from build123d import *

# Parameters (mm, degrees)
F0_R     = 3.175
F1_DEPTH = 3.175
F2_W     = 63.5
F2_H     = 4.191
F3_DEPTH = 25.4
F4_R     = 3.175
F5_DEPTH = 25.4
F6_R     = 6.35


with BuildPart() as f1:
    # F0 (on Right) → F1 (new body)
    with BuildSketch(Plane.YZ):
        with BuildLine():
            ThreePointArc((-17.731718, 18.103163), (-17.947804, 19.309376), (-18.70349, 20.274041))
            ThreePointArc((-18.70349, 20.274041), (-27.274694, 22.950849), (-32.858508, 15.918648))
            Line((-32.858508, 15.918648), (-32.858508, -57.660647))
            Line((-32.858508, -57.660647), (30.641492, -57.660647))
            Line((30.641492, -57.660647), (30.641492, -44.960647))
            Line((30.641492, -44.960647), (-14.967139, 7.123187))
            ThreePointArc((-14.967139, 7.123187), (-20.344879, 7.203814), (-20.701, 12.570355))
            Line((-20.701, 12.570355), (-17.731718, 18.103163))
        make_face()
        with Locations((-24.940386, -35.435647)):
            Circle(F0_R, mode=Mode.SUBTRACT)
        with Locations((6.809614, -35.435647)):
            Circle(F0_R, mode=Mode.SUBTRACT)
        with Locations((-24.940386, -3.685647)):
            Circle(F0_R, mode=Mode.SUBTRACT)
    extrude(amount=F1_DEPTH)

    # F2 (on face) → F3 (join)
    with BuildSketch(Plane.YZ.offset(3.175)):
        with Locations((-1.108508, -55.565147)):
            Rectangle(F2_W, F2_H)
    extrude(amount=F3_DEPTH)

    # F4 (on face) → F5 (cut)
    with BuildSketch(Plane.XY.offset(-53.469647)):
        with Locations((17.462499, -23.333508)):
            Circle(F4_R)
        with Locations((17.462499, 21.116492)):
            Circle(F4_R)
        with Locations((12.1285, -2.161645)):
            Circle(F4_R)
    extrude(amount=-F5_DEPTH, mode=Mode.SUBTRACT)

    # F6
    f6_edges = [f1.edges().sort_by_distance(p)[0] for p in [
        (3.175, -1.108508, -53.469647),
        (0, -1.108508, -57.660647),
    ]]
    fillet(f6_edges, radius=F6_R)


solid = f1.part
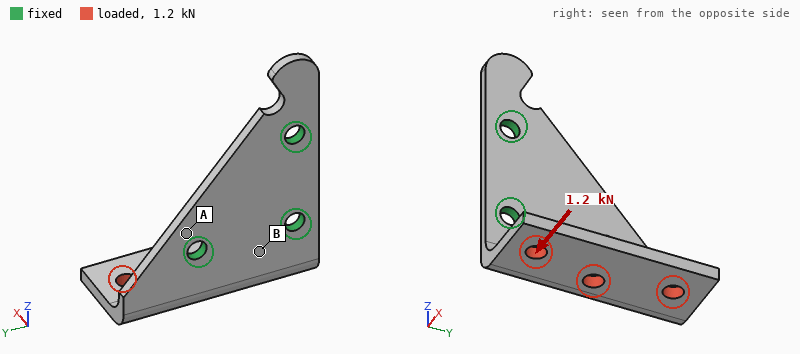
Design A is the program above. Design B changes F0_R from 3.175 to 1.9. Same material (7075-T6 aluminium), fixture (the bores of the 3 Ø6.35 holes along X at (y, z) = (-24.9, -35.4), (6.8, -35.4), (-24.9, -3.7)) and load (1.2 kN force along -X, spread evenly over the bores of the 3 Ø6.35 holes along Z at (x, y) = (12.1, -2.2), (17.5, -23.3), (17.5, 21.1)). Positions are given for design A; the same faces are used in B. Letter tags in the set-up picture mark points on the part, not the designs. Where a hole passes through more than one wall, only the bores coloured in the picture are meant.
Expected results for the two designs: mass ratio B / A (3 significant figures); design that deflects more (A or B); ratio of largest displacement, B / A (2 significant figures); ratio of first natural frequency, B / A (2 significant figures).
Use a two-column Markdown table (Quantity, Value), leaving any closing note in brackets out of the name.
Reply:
| Quantity | Value |
|---|---|
| mass ratio B / A | 1.01 |
| design that deflects more | B |
| ratio of largest displacement, B / A | 1.3 |
| ratio of first natural frequency, B / A | 0.90 |
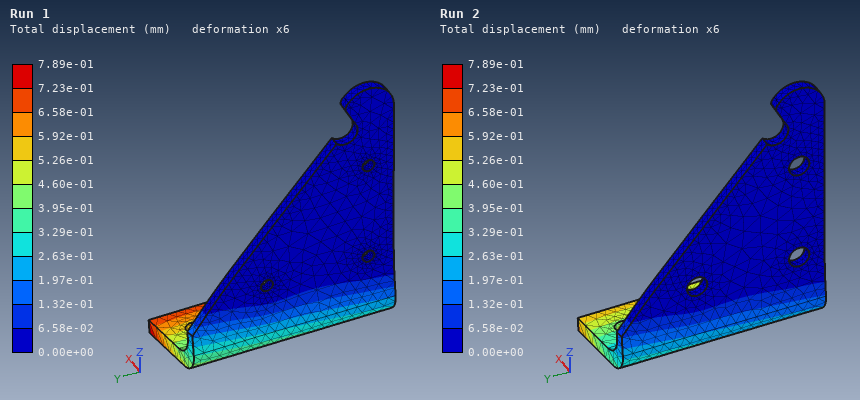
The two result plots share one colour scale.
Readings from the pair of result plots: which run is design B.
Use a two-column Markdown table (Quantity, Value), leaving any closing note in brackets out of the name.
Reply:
| Quantity | Value |
|---|---|
| which run is design B | Run 1 |
